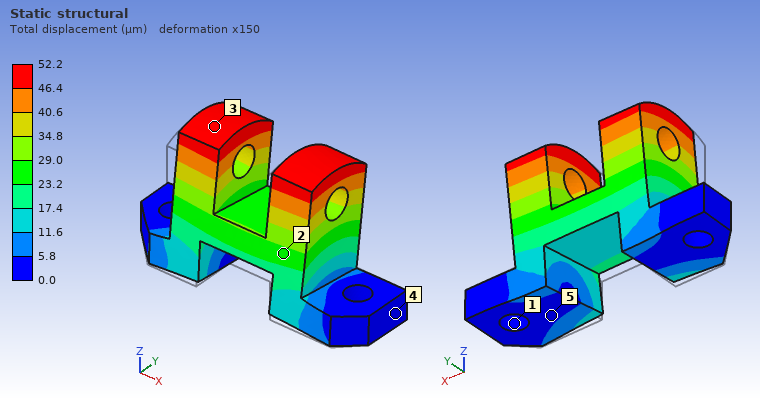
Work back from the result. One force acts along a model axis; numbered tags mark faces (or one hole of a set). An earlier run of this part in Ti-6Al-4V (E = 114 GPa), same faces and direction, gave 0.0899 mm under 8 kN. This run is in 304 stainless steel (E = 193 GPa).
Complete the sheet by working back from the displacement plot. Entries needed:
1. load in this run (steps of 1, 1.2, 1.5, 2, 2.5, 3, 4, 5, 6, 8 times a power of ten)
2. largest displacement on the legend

8 kN
52.2 µm
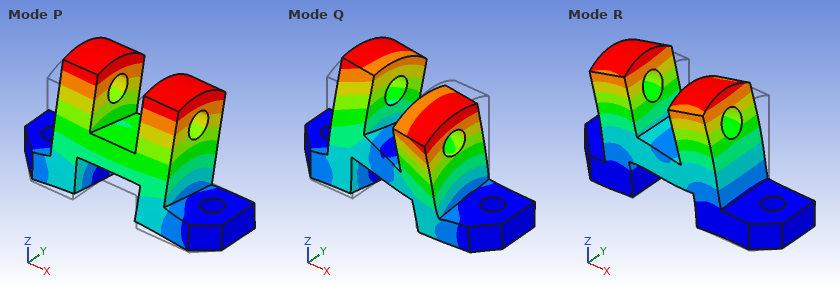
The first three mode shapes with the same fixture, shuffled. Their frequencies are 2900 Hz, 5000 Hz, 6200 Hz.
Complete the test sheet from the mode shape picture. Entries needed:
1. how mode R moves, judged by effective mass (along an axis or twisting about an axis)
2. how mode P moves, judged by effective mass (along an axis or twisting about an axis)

along X
along Y
